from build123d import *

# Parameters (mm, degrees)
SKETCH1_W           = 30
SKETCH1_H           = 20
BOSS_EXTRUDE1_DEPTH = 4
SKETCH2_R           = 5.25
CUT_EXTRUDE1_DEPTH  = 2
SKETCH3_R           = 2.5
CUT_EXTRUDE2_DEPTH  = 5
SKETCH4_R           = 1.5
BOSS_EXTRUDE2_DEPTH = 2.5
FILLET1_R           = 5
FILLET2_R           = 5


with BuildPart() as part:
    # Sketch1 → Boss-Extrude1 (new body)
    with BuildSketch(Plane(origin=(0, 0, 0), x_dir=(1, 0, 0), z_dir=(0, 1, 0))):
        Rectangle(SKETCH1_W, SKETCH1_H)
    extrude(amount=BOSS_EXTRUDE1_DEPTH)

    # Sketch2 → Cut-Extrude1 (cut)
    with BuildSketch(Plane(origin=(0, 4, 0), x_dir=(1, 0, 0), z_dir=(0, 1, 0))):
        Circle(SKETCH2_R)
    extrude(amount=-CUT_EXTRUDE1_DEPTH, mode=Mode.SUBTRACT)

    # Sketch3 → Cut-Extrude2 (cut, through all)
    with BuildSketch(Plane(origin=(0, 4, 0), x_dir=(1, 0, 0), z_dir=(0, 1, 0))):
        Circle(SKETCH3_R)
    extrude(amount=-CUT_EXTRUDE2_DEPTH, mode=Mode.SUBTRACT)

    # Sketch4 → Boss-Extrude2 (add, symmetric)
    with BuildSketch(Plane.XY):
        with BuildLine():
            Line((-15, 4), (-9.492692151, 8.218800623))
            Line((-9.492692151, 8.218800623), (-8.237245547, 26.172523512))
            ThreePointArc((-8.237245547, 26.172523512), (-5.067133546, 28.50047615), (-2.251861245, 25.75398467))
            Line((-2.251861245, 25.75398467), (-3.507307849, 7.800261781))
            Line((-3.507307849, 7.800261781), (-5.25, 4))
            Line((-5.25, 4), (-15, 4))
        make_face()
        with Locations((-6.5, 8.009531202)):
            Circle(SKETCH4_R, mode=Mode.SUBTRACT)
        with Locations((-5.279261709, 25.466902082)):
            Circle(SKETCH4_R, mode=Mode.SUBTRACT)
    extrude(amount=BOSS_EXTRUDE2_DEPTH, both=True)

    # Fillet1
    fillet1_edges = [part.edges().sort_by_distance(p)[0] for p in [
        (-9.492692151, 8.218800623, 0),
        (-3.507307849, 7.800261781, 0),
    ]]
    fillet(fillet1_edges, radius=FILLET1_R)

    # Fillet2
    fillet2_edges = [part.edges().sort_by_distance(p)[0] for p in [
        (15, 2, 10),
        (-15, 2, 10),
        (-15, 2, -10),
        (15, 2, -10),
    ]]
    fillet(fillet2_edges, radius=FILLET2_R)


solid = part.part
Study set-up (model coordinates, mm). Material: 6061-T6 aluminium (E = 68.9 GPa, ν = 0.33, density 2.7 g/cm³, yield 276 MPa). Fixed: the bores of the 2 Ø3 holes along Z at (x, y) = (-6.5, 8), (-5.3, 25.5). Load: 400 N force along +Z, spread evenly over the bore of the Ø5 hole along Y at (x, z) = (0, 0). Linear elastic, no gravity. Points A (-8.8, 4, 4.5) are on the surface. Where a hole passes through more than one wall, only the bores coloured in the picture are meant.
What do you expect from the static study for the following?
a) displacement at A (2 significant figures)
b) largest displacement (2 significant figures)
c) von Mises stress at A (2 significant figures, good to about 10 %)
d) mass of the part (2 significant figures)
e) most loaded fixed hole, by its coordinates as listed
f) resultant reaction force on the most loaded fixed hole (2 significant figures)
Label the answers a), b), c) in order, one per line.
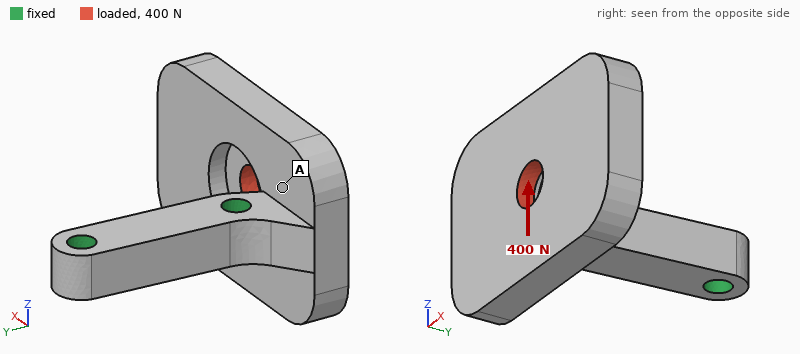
a) 17 µm
b) 97 µm
c) 24 MPa
d) 7.5 g
e) (-6.5, 8)
f) 400 N
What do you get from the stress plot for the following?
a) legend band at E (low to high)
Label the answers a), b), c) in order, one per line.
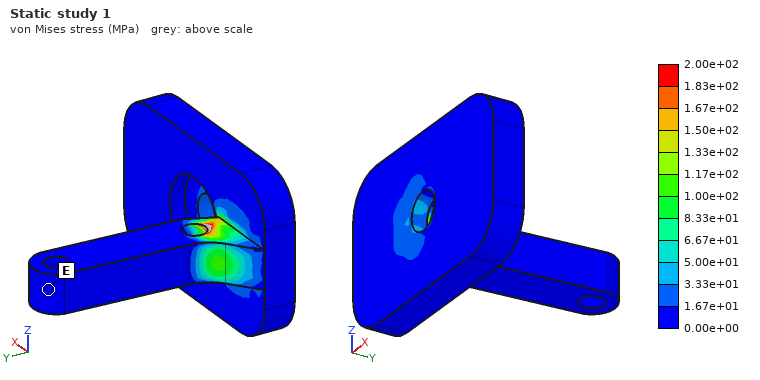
a) 0.00e+00 to 1.67e+01 MPa
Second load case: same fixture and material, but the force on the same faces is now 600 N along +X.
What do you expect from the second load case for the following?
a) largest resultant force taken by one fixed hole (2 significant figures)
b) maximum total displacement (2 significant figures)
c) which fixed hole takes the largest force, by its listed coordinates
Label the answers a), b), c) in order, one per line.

a) 640 N
b) 69 µm
c) (-6.5, 8)
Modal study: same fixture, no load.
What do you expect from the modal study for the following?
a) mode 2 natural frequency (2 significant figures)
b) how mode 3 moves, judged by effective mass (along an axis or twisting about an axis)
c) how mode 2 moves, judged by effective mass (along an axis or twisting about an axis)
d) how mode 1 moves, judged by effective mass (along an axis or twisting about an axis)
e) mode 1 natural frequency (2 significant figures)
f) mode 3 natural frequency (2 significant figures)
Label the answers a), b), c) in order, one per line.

a) 4700 Hz
b) twisting about X
c) along Z
d) along Y
e) 4000 Hz
f) 8400 Hz
